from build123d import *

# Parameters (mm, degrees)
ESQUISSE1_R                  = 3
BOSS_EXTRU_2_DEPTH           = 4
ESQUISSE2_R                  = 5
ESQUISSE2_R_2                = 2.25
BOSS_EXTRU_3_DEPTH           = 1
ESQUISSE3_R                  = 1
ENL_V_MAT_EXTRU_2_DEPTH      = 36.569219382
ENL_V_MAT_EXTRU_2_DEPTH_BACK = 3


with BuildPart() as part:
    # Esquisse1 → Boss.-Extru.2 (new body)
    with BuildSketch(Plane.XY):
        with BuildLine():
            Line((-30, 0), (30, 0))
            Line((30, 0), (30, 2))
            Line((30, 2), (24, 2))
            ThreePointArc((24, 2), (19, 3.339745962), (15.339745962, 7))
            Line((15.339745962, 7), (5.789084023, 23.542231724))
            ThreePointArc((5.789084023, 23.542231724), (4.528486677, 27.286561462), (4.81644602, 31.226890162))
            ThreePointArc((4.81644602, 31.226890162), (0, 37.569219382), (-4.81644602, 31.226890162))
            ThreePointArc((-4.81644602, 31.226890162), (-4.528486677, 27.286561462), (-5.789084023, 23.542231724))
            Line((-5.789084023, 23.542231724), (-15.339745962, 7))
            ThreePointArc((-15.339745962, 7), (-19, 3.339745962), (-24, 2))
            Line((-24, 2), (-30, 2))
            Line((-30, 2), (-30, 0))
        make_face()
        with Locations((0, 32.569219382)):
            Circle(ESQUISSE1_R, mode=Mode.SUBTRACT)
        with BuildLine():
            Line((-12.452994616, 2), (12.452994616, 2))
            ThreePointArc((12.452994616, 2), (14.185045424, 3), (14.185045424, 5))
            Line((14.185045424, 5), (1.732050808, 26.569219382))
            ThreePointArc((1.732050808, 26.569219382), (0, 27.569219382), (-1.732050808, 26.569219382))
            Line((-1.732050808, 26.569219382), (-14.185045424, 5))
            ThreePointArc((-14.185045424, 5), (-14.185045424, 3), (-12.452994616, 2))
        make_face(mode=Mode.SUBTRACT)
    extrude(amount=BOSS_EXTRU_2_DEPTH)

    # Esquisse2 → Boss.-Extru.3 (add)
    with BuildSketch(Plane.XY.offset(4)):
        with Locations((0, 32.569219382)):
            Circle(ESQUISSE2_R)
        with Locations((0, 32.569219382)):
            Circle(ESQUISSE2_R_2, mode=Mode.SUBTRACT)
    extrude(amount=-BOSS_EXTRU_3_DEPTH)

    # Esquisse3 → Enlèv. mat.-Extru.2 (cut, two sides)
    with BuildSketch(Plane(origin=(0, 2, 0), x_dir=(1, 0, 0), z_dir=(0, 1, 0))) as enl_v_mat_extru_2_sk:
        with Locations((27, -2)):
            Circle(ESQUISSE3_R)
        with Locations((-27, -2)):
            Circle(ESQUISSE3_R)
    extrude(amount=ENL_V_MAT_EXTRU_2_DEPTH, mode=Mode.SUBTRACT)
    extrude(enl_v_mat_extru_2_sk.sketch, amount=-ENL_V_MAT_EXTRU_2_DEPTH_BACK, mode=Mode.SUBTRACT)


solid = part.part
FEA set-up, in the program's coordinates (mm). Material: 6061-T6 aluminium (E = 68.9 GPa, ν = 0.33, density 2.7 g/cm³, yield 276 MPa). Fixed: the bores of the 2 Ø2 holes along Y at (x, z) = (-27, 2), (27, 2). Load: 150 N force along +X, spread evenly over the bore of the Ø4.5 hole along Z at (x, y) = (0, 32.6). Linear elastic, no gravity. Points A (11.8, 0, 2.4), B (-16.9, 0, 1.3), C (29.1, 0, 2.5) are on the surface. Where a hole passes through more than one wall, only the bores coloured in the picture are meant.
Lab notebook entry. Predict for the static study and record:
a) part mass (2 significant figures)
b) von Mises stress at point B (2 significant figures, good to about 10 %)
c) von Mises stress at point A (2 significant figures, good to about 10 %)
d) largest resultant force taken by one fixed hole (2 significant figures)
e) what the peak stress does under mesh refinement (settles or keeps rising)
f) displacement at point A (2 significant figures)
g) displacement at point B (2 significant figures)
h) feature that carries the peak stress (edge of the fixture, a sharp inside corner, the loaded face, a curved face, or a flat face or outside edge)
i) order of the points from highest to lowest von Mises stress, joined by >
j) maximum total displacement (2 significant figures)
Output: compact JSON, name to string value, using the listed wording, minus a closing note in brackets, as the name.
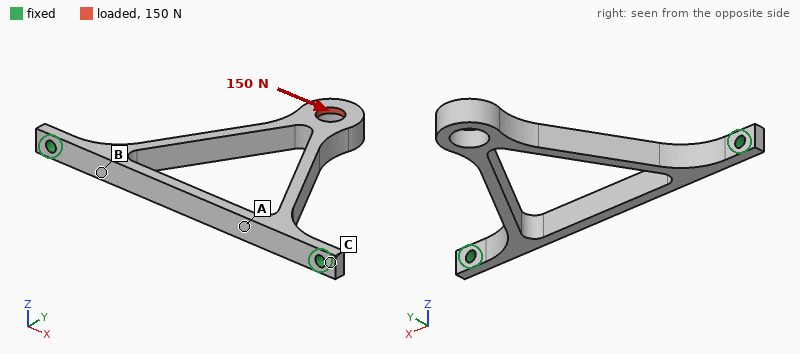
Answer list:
{"part mass": "3.4 g", "von Mises stress at point B": "38 MPa", "von Mises stress at point A": "88 MPa", "largest resultant force taken by one fixed hole": "130 N", "what the peak stress does under mesh refinement": "keeps rising", "displacement at point A": "0.059 mm", "displacement at point B": "0.045 mm", "feature that carries the peak stress": "edge of the fixture", "order of the points from highest to lowest von Mises stress, joined by >": "A > B > C", "maximum total displacement": "0.15 mm"}
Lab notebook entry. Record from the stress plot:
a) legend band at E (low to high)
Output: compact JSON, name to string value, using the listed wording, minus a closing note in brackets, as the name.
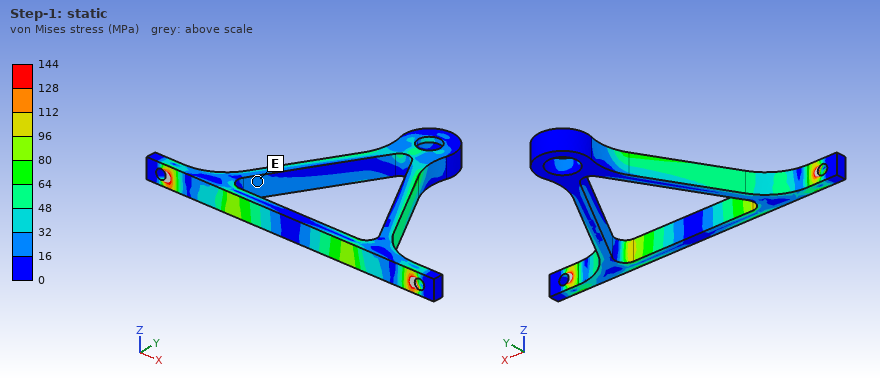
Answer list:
{"legend band at E": "16 to 32 MPa"}
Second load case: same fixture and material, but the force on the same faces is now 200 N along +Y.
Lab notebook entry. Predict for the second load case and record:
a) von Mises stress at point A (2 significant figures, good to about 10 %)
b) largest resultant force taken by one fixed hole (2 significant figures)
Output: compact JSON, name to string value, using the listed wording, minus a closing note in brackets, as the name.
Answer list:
{"von Mises stress at point A": "33 MPa", "largest resultant force taken by one fixed hole": "120 N"}
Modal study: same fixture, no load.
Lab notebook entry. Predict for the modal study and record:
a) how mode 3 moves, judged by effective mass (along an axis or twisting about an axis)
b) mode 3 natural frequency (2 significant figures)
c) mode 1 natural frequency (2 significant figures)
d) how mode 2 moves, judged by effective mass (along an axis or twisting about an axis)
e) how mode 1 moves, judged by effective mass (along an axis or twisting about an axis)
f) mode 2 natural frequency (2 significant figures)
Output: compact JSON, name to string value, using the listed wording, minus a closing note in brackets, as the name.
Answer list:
{"how mode 3 moves, judged by effective mass": "twisting about Z", "mode 3 natural frequency": "5000 Hz", "mode 1 natural frequency": "1100 Hz", "how mode 2 moves, judged by effective mass": "along Y", "how mode 1 moves, judged by effective mass": "along Z", "mode 2 natural frequency": "3800 Hz"}
